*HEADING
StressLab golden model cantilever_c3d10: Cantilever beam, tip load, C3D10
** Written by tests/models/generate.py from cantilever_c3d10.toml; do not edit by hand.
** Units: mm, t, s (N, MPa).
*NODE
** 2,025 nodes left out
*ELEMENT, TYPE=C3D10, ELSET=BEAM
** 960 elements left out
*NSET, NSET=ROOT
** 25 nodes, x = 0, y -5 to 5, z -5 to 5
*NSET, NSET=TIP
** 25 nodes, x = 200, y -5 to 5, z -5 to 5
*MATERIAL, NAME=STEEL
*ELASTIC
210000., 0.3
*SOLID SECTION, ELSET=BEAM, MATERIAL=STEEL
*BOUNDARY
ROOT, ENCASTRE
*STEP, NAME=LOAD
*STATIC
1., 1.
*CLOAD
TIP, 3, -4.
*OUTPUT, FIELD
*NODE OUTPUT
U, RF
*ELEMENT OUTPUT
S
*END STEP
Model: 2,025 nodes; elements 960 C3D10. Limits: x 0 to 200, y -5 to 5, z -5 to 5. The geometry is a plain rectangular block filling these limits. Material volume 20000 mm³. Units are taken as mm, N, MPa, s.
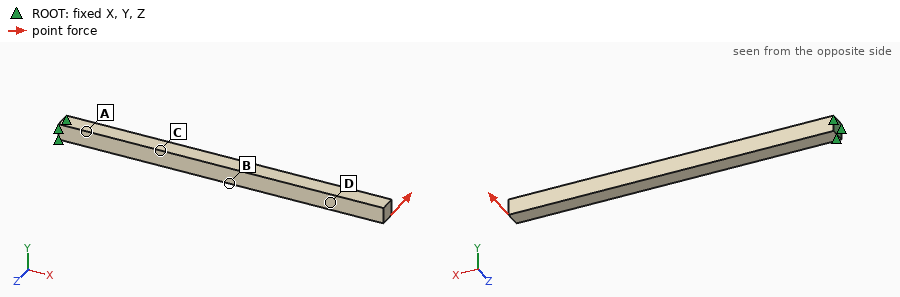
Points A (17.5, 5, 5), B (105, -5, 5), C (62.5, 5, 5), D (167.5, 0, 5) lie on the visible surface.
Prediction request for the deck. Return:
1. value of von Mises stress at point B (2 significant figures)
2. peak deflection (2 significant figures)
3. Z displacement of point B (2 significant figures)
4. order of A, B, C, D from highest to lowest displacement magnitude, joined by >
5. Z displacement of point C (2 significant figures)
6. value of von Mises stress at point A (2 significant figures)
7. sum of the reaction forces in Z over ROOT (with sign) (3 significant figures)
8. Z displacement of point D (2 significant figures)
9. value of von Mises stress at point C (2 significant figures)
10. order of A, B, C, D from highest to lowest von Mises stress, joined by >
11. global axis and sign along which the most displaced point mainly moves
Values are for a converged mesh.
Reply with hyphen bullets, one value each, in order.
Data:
- 57 MPa
- 1.5 mm
- -0.52 mm
- D > B > C > A
- -0.20 mm
- 110 MPa
- 100 N
- -1.2 mm
- 83 MPa
- A > C > B > D
- -Z
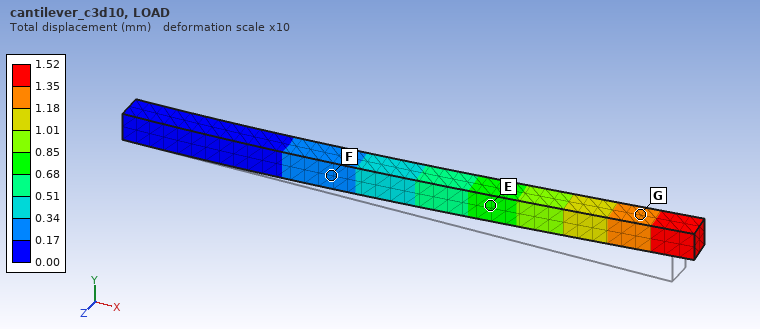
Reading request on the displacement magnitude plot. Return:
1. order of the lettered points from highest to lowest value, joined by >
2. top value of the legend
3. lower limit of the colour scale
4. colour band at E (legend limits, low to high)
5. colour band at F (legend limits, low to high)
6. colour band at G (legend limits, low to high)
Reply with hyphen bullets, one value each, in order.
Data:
- G > E > F
- 1.52 mm
- 0.00 mm
- 0.68 to 0.85 mm
- 0.17 to 0.34 mm
- 1.18 to 1.35 mm
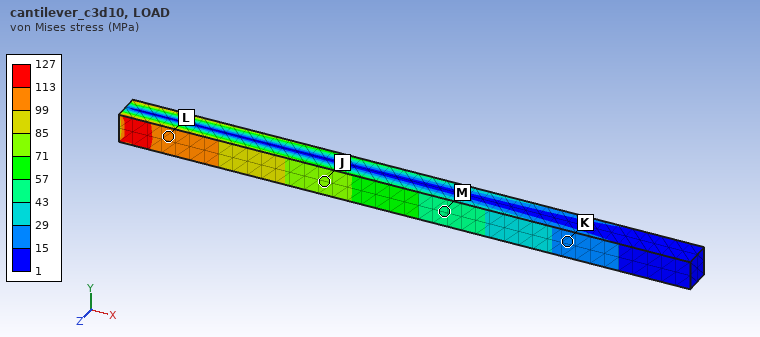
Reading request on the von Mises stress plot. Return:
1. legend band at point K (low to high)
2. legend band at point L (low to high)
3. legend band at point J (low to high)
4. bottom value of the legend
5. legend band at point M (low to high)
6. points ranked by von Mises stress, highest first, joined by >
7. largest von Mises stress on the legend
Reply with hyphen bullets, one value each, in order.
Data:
- 15 to 29 MPa
- 99 to 113 MPa
- 71 to 85 MPa
- 1 MPa
- 43 to 57 MPa
- L > J > M > K
- 127 MPa
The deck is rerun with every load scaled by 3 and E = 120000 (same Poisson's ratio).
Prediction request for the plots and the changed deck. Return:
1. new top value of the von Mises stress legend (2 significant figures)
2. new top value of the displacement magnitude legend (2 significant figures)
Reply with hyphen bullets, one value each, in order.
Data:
- 380 MPa
- 8.0 mm
